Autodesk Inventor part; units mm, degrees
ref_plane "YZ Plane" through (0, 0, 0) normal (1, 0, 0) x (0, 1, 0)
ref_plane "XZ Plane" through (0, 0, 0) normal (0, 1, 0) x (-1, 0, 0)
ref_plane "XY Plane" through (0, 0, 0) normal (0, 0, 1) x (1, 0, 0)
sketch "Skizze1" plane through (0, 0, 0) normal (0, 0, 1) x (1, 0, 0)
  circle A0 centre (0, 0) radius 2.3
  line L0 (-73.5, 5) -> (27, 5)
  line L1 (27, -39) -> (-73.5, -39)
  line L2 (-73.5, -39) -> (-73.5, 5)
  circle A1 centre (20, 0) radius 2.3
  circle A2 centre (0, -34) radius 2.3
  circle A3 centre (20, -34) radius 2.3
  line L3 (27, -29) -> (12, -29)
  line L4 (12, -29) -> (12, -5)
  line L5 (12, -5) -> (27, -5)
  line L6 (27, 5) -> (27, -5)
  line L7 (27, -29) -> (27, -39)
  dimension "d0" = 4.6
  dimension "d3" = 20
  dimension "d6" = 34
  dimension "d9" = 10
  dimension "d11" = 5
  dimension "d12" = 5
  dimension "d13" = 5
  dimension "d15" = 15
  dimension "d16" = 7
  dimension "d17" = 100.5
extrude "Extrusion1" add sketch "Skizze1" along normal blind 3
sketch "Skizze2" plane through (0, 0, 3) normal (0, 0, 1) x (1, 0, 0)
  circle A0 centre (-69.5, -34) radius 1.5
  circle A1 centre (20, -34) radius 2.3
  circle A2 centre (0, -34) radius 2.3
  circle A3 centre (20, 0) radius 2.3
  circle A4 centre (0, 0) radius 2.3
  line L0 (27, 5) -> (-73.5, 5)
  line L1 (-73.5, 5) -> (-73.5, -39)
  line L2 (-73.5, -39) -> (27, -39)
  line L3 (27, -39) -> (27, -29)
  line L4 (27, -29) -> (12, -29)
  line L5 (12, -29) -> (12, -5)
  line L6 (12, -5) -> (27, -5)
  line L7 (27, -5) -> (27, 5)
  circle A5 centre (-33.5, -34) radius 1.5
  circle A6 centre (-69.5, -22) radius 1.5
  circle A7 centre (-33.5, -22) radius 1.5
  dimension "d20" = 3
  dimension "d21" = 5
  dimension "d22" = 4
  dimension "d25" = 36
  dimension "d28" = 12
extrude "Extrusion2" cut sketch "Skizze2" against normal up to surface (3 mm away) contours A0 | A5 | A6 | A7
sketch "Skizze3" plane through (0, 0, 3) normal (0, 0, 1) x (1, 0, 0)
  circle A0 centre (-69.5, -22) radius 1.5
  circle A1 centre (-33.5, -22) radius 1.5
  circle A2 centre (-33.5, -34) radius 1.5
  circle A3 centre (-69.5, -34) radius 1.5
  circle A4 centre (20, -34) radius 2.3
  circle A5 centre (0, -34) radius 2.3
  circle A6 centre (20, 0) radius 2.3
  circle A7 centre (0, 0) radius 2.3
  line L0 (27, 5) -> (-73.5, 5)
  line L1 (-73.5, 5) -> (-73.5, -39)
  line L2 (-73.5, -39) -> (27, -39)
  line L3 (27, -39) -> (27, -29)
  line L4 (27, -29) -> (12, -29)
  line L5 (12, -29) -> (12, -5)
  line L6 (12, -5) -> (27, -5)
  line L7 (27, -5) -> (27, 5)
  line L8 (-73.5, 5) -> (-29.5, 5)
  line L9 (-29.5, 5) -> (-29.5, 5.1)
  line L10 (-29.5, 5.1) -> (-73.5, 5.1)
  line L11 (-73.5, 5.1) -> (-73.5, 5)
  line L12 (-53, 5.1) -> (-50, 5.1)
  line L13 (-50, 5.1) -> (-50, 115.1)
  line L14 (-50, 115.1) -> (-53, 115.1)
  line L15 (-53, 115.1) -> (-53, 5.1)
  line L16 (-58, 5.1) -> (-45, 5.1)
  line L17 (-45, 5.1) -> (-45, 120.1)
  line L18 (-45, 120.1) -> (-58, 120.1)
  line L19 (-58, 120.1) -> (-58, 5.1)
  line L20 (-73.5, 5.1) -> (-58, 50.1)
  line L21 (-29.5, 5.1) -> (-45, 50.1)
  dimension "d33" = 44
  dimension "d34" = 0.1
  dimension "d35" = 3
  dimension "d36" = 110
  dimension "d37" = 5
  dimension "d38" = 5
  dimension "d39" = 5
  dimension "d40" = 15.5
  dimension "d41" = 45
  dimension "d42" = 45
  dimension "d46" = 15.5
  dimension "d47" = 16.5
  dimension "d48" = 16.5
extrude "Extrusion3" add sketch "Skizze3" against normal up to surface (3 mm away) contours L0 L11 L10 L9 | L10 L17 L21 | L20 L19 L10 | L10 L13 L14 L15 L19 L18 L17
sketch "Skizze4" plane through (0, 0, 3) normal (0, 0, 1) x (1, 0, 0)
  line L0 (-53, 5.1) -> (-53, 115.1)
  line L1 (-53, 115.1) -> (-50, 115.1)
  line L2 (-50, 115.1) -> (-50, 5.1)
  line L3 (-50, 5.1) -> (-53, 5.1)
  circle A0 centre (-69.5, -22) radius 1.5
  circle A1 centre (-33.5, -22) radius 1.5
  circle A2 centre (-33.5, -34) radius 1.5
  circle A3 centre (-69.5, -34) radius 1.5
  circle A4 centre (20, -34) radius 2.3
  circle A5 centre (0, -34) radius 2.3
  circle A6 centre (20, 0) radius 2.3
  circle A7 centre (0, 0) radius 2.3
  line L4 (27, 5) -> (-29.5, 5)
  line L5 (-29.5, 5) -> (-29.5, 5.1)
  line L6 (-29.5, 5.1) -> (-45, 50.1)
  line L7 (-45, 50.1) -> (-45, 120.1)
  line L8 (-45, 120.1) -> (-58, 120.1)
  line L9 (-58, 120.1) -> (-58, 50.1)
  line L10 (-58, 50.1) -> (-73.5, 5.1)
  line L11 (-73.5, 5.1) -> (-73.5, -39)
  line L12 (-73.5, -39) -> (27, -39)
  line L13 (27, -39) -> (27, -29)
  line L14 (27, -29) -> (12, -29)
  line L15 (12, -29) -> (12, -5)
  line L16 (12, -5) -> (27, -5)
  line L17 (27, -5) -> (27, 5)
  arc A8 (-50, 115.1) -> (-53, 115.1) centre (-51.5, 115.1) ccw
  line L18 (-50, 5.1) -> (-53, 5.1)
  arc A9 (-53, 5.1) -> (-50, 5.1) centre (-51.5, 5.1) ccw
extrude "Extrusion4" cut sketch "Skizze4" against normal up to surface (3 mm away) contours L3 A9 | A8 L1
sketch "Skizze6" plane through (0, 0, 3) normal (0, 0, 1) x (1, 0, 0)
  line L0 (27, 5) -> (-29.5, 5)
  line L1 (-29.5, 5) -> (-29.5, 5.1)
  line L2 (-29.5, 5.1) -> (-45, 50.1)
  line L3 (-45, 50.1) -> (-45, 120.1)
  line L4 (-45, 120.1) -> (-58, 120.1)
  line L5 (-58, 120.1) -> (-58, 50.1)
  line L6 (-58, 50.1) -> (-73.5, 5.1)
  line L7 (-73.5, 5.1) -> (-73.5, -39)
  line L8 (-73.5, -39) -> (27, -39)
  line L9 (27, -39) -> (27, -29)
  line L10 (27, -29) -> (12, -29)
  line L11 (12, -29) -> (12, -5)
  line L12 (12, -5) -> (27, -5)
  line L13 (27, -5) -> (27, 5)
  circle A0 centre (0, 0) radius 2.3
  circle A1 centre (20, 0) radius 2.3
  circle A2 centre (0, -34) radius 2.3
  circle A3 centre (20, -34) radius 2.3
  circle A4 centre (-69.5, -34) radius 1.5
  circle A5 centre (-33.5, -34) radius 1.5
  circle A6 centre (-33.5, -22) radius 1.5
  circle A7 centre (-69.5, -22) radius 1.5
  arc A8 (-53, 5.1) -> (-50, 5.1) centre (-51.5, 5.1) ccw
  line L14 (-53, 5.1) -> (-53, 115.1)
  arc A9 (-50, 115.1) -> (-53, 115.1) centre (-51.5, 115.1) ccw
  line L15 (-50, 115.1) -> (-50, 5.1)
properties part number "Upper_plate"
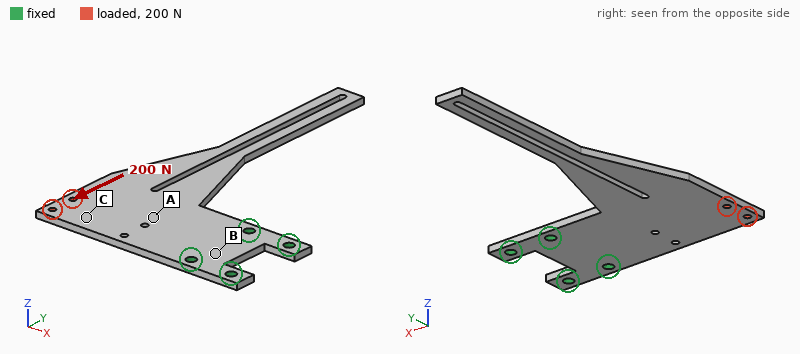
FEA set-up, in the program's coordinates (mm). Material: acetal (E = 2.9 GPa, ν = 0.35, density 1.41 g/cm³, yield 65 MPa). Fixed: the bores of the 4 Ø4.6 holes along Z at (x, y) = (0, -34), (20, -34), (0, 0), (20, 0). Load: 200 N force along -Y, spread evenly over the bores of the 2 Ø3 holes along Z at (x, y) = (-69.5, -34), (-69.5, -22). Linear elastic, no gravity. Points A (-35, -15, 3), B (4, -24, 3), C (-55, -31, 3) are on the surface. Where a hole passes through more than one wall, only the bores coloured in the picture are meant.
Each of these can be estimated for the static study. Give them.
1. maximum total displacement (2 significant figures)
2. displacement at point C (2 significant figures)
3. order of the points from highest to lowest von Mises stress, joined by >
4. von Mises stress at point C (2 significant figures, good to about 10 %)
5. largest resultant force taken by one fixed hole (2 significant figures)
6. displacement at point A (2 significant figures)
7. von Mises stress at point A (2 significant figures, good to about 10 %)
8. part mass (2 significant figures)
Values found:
1.2 mm
0.36 mm
A > C > B
2.8 MPa
390 N
0.17 mm
4.4 MPa
25 g
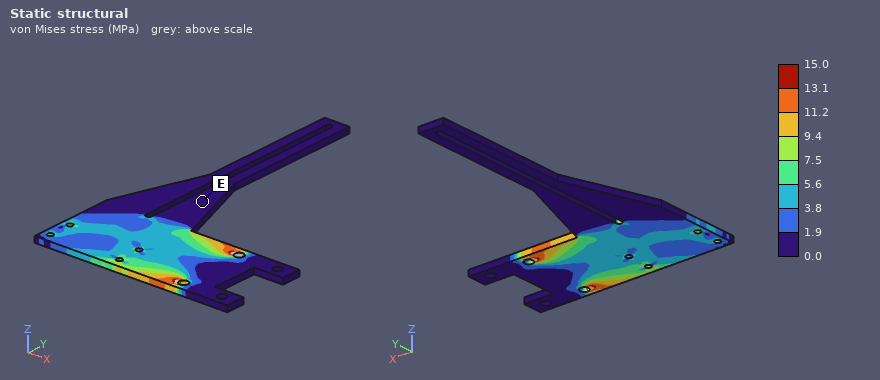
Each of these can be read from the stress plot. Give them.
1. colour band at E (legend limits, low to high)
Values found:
0.0 to 1.9 MPa
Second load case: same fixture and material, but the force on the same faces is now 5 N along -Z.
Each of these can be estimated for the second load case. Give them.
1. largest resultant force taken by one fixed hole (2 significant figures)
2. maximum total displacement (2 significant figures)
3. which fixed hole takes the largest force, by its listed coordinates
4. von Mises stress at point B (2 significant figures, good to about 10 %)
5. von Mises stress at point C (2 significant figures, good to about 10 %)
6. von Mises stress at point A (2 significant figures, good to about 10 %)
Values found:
6.4 N
2.2 mm
(0, -34)
1.6 MPa
1.4 MPa
2.6 MPa
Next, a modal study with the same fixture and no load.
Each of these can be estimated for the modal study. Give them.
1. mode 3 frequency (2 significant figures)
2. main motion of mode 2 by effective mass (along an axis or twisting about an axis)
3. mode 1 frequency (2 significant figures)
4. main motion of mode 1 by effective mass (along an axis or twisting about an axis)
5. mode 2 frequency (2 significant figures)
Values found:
240 Hz
along Z
52 Hz
along Z
110 Hz
